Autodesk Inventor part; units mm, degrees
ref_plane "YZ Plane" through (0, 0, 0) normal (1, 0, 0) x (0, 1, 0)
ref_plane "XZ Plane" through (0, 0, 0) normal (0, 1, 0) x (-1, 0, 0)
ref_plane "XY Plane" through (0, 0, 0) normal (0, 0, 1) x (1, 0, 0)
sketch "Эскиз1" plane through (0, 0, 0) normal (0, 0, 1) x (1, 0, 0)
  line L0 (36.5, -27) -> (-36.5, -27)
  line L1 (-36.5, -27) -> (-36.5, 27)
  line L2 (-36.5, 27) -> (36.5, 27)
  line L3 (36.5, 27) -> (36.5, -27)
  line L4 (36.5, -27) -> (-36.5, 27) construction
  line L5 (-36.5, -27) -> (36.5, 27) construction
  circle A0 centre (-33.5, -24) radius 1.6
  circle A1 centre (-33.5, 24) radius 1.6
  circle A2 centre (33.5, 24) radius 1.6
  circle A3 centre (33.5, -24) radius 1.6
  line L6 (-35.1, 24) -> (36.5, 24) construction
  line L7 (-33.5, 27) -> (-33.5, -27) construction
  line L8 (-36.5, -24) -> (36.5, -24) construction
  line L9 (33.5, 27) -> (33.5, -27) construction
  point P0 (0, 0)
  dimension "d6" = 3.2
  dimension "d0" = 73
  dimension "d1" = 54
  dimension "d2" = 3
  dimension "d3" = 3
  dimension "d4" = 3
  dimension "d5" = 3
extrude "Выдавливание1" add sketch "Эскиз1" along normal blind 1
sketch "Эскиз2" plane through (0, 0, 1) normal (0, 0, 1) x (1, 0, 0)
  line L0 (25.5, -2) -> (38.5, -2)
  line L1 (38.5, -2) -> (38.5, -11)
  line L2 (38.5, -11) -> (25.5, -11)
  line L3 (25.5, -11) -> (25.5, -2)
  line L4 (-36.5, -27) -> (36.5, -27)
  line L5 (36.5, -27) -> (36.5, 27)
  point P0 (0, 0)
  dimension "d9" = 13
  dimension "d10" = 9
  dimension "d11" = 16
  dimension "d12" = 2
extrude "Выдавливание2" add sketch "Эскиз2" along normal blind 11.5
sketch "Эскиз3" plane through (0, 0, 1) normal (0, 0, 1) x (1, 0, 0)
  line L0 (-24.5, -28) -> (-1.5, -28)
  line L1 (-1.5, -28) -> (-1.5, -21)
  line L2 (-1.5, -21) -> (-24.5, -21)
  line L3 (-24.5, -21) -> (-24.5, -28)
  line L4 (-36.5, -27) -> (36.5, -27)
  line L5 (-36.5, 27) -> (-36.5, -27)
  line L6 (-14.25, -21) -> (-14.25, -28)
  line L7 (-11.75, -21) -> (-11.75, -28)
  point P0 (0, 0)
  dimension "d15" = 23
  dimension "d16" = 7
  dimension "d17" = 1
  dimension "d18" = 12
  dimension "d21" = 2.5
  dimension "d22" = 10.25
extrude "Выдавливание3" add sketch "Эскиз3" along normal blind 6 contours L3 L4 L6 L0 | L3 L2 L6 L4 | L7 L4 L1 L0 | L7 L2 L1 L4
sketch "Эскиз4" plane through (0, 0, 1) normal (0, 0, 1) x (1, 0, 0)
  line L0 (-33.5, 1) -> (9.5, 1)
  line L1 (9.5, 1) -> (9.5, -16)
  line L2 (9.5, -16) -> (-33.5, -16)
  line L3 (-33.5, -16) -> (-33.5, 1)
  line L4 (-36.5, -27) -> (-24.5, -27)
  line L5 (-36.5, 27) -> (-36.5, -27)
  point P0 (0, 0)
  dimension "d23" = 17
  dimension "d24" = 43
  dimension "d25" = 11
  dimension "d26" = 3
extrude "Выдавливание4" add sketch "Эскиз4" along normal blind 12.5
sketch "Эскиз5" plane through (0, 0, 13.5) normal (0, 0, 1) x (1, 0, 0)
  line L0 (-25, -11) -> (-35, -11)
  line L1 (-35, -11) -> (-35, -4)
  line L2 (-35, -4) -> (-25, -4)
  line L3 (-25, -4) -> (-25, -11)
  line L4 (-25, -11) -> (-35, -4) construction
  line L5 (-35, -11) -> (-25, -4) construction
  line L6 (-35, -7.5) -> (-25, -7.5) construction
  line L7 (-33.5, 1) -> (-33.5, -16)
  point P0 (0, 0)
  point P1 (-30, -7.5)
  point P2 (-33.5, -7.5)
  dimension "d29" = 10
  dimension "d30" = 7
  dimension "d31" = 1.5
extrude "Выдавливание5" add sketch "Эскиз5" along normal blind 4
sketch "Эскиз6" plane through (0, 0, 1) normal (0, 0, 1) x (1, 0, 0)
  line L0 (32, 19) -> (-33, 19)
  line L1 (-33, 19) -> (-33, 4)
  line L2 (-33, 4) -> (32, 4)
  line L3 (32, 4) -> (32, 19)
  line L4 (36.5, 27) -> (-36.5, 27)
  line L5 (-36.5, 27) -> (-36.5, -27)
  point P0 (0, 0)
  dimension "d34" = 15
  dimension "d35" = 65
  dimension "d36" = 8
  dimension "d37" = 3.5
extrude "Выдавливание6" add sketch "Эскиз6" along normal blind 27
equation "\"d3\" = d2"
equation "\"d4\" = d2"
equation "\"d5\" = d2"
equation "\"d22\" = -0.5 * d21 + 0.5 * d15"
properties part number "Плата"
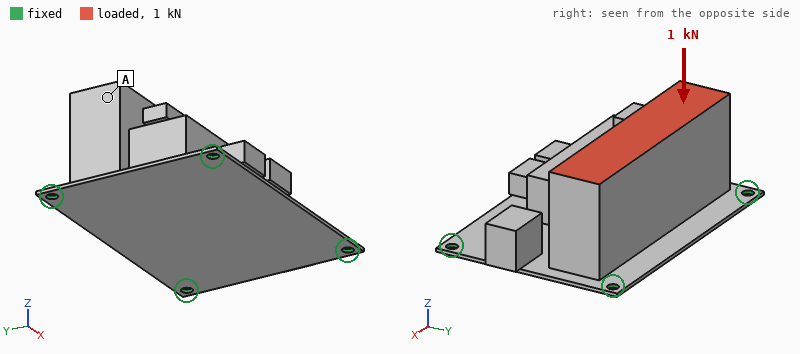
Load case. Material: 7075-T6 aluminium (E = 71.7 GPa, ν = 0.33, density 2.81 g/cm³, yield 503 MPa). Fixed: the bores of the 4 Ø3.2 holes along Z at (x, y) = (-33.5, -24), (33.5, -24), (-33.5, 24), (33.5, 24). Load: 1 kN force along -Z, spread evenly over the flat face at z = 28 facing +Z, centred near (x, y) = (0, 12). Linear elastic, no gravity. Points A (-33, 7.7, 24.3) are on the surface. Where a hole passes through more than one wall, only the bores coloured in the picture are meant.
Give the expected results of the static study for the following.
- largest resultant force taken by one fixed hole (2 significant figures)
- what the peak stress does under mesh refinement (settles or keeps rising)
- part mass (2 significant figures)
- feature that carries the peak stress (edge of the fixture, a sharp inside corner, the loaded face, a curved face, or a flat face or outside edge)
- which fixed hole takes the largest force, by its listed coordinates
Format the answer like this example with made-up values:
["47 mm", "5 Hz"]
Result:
["500 N", "keeps rising", "120 g", "edge of the fixture", "(33.5, 24)"]
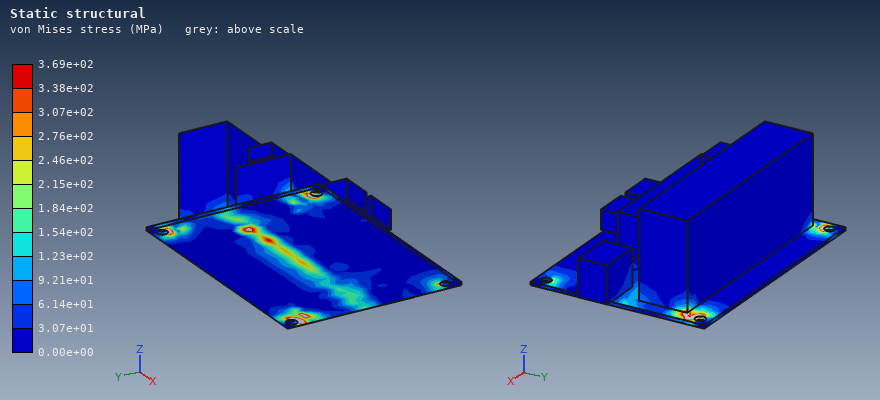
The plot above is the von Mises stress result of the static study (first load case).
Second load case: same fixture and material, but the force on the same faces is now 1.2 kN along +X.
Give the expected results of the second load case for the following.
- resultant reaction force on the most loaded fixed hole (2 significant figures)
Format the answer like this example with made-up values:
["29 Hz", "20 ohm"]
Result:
["700 N"]
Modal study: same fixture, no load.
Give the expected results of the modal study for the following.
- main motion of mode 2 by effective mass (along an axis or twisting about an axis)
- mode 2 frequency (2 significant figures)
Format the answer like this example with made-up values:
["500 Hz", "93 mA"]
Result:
["along Z", "1800 Hz"]
